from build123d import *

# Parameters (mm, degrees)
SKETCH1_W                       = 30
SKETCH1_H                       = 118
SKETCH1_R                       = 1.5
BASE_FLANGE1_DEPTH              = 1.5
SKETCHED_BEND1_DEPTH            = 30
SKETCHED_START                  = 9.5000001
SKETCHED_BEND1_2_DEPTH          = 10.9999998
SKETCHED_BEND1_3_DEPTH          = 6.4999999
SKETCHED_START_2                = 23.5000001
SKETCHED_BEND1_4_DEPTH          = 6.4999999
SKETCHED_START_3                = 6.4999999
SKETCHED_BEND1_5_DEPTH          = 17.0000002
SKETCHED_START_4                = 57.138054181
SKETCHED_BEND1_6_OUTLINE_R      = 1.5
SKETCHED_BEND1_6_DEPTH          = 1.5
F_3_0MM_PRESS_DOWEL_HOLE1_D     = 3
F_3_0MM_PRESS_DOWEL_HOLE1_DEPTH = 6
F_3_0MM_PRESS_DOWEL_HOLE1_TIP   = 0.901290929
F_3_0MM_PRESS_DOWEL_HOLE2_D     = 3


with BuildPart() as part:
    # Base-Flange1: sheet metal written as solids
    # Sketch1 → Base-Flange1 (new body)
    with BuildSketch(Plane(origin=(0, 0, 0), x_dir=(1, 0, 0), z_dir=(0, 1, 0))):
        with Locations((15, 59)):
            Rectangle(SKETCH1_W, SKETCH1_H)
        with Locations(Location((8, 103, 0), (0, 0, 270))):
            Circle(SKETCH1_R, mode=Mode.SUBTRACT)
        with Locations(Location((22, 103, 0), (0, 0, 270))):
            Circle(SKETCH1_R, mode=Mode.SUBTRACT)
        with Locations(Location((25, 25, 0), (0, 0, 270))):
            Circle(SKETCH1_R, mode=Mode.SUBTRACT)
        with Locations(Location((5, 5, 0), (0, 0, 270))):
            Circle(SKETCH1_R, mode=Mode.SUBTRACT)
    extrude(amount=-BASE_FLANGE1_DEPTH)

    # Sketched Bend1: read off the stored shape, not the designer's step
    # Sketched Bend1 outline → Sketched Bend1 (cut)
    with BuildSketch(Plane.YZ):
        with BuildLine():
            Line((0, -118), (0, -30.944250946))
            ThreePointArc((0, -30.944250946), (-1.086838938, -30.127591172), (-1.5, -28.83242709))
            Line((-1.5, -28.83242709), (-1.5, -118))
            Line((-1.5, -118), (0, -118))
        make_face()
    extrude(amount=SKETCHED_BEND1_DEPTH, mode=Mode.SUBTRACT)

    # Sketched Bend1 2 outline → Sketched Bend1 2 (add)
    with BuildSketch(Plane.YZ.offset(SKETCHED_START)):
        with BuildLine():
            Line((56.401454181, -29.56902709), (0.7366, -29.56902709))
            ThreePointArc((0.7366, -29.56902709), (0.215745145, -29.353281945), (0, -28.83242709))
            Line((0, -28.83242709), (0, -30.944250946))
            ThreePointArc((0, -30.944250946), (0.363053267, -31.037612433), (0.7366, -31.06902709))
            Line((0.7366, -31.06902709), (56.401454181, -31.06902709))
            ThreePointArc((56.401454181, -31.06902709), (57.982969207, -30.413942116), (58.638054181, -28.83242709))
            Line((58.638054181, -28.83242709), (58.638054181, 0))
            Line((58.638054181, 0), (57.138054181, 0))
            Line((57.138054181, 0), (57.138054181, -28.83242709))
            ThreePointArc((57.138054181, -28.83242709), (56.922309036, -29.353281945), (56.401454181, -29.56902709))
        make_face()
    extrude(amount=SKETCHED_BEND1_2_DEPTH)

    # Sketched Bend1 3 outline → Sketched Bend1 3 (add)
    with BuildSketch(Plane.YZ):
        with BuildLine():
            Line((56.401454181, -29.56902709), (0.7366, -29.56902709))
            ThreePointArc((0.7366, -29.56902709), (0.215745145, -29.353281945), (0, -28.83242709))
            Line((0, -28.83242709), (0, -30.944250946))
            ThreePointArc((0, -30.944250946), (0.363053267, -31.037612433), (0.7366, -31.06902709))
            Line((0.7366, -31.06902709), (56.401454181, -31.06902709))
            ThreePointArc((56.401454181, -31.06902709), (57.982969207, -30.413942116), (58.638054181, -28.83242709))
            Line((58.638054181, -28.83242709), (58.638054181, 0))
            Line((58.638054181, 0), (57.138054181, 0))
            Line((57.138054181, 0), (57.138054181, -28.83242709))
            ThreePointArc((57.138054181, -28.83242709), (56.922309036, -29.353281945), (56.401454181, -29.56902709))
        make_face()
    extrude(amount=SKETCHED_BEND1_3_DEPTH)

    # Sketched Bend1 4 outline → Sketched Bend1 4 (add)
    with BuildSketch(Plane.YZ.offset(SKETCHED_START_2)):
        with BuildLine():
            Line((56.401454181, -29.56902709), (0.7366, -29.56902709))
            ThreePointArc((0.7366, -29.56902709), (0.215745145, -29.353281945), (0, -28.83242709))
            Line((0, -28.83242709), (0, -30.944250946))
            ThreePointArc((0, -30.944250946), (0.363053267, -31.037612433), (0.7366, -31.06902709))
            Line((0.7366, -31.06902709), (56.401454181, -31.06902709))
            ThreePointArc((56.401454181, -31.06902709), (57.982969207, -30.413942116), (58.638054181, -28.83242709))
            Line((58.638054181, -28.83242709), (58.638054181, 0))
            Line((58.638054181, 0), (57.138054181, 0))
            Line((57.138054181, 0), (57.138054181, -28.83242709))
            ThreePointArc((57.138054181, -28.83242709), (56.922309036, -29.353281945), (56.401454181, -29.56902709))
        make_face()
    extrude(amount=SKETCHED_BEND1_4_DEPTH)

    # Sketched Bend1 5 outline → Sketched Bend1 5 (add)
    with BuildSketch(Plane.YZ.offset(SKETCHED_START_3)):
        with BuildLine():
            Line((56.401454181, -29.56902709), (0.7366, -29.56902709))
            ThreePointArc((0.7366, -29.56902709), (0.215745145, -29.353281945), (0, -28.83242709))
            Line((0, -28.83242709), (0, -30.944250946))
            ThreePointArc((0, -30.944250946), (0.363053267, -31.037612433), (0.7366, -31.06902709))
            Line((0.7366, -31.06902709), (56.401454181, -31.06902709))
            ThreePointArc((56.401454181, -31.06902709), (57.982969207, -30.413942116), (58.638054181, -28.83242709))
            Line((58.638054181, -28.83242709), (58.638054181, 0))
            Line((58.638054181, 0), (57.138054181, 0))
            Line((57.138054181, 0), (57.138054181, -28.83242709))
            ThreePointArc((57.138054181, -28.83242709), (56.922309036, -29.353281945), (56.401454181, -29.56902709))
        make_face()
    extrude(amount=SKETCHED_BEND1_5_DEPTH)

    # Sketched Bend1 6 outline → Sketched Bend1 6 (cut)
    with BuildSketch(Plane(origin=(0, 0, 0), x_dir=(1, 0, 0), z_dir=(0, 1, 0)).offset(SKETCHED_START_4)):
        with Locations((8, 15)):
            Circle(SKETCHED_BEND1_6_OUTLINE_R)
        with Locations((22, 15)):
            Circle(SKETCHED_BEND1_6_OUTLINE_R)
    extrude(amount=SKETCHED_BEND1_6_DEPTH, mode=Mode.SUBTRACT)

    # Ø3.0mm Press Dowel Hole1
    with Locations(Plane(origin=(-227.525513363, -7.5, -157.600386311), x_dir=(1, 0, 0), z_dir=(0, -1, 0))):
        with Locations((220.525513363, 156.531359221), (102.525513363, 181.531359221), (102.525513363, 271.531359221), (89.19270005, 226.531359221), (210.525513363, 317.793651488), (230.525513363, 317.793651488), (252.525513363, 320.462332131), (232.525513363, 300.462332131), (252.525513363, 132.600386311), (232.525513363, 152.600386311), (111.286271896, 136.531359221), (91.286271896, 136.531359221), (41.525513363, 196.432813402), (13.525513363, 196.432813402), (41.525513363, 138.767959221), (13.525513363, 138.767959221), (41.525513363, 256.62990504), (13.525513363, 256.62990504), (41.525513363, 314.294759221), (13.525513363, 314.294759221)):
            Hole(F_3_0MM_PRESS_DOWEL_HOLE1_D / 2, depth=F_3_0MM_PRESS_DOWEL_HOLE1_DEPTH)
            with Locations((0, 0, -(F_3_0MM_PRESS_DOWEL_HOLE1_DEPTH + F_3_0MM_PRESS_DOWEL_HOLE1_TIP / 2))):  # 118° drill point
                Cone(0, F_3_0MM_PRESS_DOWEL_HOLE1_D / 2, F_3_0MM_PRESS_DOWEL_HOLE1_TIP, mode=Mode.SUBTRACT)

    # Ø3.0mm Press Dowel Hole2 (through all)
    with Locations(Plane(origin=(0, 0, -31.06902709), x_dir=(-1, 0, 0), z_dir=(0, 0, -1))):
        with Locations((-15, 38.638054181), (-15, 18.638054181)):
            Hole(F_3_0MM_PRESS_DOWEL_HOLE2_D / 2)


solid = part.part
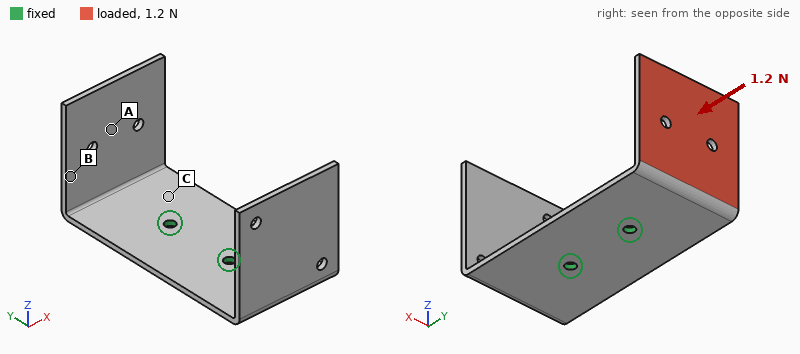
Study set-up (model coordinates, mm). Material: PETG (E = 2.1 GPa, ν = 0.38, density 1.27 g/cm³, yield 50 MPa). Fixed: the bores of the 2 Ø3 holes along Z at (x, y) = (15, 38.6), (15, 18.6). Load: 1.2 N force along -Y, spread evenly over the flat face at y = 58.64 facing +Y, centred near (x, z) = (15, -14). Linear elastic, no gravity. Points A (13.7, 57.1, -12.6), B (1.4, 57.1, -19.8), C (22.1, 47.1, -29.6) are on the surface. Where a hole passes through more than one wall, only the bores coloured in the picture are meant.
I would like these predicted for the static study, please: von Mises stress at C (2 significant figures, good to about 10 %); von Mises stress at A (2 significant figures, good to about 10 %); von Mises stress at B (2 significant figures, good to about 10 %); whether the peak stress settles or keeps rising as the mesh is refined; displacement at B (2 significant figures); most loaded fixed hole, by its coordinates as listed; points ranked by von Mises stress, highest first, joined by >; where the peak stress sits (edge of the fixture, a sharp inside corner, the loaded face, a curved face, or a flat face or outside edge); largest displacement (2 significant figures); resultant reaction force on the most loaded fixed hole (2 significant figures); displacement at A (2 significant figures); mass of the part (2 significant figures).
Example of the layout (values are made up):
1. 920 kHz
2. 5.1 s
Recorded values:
1. 1.6 MPa
2. 0.31 MPa
3. 0.72 MPa
4. keeps rising
5. 0.30 mm
6. (15, 38.6)
7. C > B > A
8. edge of the fixture
9. 0.85 mm
10. 0.97 N
11. 0.48 mm
12. 6.7 g
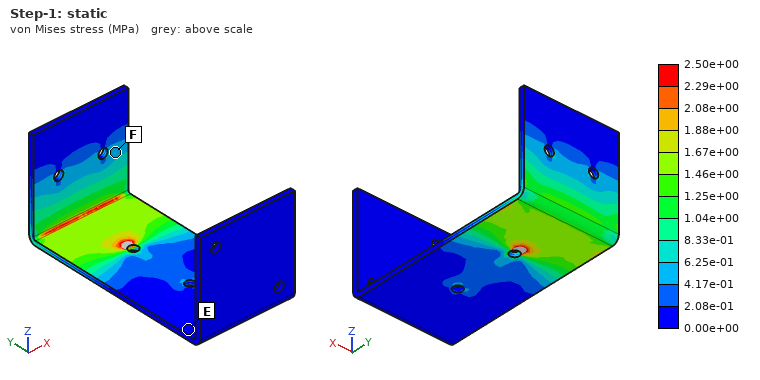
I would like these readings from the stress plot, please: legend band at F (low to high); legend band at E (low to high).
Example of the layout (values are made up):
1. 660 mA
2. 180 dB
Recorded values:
1. 4.17e-01 to 6.25e-01 MPa
2. 0.00e+00 to 2.08e-01 MPa
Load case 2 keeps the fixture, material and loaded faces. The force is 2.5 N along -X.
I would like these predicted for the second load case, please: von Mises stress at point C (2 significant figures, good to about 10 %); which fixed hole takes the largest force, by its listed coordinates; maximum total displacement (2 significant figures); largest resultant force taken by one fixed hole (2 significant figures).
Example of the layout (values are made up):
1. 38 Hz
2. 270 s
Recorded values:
1. 2.1 MPa
2. (15, 38.6)
3. 0.87 mm
4. 4.7 N
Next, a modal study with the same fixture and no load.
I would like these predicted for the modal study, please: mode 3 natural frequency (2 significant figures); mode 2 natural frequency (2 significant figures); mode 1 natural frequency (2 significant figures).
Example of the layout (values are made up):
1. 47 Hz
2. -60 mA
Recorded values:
1. 240 Hz
2. 170 Hz
3. 160 Hz
